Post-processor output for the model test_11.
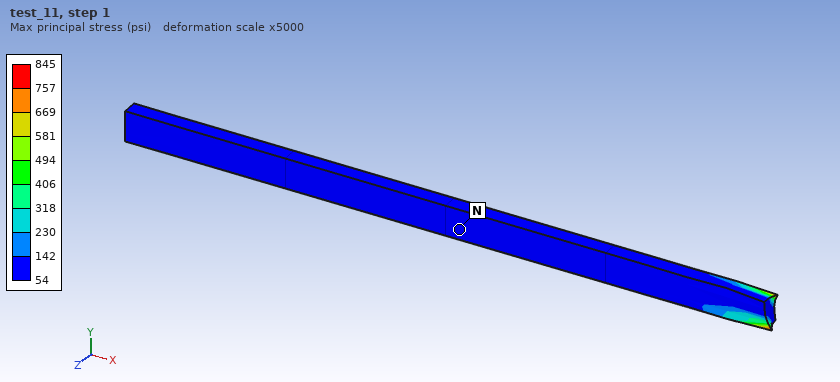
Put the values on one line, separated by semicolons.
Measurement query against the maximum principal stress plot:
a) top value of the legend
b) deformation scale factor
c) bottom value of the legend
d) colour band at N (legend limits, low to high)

845 psi; 5000; 54 psi; 54 to 142 psi
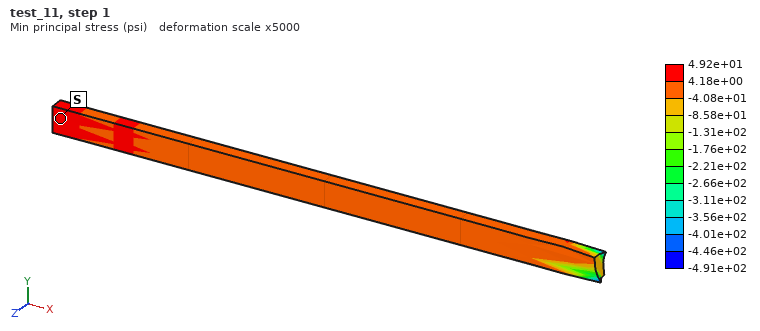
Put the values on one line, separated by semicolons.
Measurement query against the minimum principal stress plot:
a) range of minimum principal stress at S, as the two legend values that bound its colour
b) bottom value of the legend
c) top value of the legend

4.18e+00 to 4.92e+01 psi; -4.91e+02 psi; 4.92e+01 psi
